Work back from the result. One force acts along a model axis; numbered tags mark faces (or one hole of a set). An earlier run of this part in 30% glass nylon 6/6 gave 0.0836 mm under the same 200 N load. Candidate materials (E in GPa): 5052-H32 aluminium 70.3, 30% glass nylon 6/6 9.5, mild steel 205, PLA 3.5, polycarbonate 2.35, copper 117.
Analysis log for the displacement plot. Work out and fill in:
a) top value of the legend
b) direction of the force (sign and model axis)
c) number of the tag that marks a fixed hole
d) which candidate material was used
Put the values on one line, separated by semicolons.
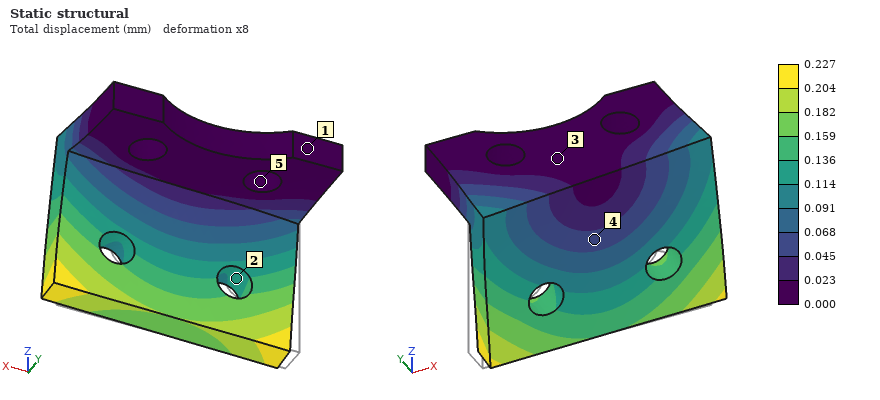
0.227 mm; +X; 5; PLA
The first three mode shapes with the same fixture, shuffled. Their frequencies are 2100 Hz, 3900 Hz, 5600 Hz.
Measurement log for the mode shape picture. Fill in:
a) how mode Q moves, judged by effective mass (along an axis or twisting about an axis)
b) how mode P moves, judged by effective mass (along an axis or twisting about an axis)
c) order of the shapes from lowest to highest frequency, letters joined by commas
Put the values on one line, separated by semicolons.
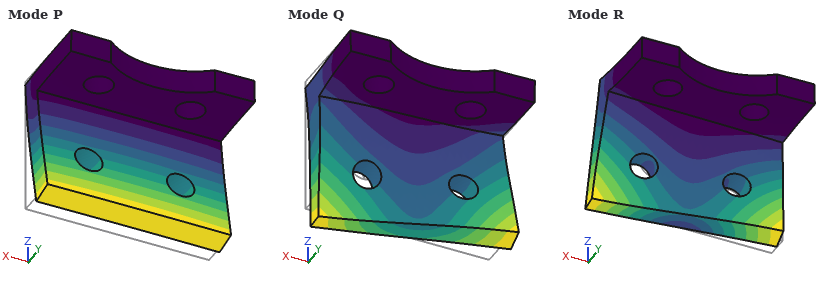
along X; along Y; P, R, Q
